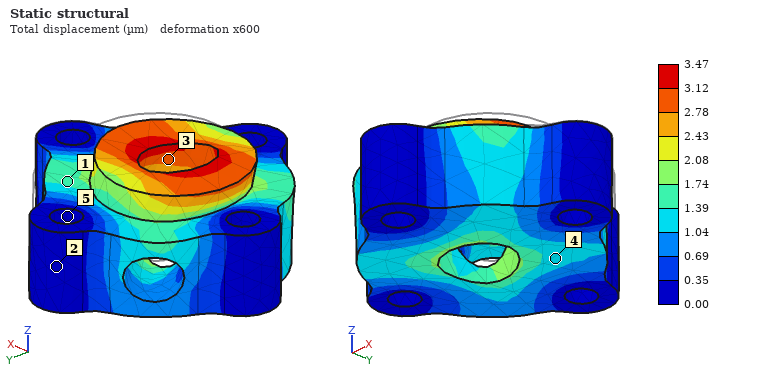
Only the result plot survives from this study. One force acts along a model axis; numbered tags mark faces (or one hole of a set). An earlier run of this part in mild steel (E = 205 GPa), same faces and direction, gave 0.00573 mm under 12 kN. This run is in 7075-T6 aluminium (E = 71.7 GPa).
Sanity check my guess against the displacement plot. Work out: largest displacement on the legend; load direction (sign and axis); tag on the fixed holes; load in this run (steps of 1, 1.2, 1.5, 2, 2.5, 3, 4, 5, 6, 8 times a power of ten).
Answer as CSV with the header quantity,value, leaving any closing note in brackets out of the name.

quantity,value
largest displacement on the legend,3.47 µm
load direction,-X
tag on the fixed holes,5
load in this run,2.5 kN
